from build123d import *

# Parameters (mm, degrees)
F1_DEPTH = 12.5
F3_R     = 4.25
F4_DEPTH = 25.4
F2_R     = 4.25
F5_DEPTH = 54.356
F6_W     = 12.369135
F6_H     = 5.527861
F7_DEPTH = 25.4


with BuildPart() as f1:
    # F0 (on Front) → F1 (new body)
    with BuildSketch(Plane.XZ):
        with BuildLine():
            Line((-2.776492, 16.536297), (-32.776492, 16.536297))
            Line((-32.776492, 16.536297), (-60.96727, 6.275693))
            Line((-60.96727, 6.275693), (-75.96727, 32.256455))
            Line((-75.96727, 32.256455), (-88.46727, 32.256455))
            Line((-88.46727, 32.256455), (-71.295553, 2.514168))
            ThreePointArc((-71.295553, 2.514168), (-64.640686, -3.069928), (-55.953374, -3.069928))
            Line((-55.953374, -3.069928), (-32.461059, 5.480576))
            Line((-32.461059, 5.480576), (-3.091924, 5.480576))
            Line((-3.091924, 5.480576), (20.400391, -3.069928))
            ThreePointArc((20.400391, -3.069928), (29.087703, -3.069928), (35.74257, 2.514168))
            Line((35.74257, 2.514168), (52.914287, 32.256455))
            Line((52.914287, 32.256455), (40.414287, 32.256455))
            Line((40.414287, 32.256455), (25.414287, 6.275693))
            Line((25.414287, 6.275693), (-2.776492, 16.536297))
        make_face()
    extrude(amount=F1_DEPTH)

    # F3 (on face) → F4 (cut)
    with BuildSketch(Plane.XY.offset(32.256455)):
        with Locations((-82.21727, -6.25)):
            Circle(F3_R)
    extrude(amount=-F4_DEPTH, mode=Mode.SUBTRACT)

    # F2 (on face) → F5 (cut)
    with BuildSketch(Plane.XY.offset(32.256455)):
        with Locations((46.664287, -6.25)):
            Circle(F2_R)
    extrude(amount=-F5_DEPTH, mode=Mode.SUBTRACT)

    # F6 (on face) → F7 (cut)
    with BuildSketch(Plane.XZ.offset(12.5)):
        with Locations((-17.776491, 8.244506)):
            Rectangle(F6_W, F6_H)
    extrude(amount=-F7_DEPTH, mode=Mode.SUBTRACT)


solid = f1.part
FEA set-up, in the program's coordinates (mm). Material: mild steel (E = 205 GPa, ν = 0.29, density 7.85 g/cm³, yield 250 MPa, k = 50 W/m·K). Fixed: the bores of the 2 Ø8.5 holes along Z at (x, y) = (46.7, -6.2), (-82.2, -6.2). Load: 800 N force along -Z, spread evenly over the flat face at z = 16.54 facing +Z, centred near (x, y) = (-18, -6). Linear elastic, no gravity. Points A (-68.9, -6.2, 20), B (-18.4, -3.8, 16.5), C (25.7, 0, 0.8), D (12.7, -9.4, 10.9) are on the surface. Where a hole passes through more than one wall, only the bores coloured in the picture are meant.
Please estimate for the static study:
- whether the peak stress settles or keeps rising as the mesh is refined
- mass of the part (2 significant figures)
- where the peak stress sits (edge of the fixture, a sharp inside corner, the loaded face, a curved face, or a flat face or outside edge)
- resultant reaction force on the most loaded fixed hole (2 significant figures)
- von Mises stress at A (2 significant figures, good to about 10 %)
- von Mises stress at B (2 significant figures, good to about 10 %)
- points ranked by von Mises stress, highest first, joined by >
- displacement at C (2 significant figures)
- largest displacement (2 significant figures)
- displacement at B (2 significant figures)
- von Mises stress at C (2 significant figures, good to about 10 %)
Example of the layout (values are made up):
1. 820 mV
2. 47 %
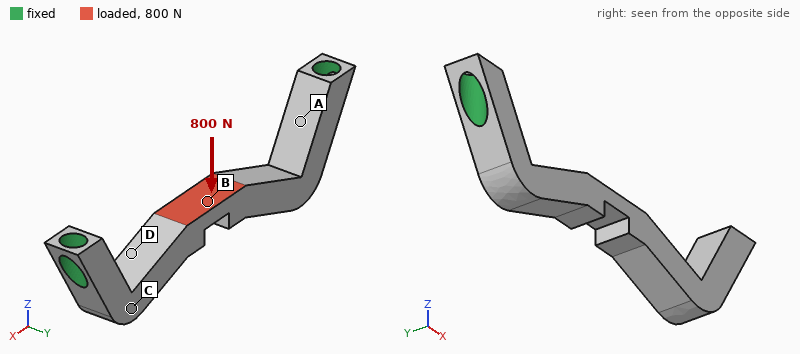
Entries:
1. keeps rising
2. 160 g
3. edge of the fixture
4. 640 N
5. 57 MPa
6. 77 MPa
7. B > A > C > D
8. 18 µm
9. 58 µm
10. 57 µm
11. 15 MPa
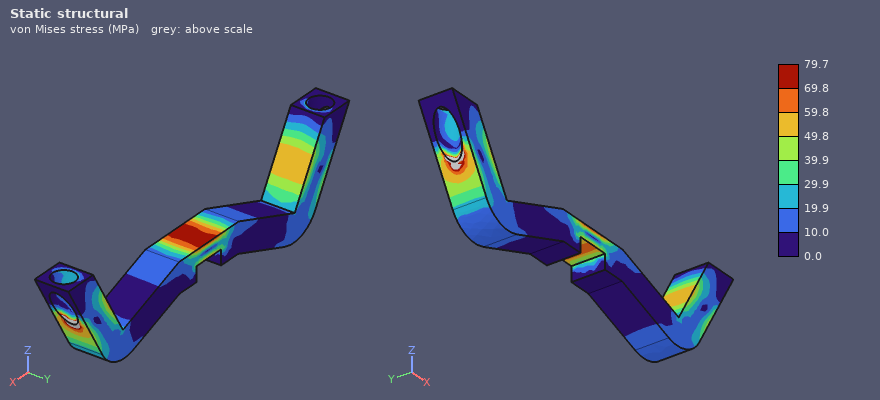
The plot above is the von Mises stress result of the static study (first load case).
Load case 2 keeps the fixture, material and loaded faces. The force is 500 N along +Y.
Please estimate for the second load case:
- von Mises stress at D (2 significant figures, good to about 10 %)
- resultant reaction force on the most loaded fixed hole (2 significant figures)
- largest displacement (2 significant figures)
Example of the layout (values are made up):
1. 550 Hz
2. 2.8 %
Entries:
1. 16 MPa
2. 250 N
3. 34 µm
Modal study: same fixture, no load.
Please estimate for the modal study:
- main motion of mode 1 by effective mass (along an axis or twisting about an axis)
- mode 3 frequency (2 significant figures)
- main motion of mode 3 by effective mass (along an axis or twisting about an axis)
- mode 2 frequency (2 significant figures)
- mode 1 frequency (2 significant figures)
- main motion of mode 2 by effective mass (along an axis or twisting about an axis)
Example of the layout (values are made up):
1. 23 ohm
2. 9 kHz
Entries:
1. along Z
2. 6600 Hz
3. along X
4. 3100 Hz
5. 2800 Hz
6. along Y
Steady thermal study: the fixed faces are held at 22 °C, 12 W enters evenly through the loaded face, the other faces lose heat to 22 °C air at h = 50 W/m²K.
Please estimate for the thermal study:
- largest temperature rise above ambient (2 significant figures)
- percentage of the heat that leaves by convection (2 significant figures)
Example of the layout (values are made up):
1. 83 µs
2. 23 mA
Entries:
1. 41 K
2. 46 %
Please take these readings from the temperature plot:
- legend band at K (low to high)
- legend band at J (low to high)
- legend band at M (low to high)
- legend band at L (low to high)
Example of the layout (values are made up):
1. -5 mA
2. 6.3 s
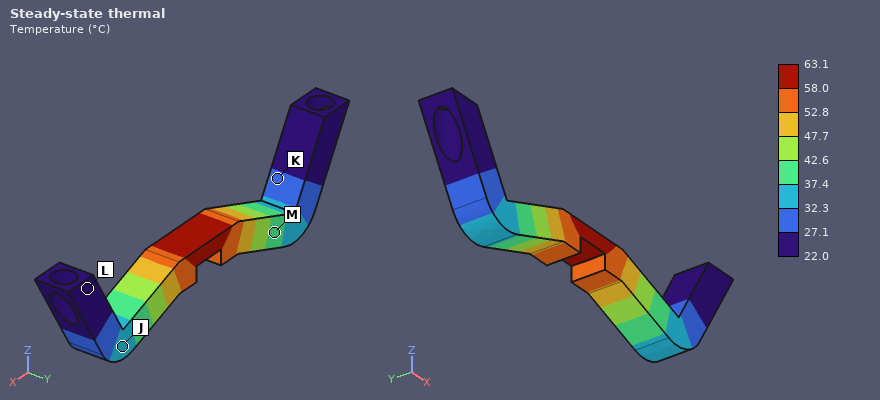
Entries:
1. 27.1 to 32.3 °C
2. 32.3 to 37.4 °C
3. 37.4 to 42.6 °C
4. 22.0 to 27.1 °C
